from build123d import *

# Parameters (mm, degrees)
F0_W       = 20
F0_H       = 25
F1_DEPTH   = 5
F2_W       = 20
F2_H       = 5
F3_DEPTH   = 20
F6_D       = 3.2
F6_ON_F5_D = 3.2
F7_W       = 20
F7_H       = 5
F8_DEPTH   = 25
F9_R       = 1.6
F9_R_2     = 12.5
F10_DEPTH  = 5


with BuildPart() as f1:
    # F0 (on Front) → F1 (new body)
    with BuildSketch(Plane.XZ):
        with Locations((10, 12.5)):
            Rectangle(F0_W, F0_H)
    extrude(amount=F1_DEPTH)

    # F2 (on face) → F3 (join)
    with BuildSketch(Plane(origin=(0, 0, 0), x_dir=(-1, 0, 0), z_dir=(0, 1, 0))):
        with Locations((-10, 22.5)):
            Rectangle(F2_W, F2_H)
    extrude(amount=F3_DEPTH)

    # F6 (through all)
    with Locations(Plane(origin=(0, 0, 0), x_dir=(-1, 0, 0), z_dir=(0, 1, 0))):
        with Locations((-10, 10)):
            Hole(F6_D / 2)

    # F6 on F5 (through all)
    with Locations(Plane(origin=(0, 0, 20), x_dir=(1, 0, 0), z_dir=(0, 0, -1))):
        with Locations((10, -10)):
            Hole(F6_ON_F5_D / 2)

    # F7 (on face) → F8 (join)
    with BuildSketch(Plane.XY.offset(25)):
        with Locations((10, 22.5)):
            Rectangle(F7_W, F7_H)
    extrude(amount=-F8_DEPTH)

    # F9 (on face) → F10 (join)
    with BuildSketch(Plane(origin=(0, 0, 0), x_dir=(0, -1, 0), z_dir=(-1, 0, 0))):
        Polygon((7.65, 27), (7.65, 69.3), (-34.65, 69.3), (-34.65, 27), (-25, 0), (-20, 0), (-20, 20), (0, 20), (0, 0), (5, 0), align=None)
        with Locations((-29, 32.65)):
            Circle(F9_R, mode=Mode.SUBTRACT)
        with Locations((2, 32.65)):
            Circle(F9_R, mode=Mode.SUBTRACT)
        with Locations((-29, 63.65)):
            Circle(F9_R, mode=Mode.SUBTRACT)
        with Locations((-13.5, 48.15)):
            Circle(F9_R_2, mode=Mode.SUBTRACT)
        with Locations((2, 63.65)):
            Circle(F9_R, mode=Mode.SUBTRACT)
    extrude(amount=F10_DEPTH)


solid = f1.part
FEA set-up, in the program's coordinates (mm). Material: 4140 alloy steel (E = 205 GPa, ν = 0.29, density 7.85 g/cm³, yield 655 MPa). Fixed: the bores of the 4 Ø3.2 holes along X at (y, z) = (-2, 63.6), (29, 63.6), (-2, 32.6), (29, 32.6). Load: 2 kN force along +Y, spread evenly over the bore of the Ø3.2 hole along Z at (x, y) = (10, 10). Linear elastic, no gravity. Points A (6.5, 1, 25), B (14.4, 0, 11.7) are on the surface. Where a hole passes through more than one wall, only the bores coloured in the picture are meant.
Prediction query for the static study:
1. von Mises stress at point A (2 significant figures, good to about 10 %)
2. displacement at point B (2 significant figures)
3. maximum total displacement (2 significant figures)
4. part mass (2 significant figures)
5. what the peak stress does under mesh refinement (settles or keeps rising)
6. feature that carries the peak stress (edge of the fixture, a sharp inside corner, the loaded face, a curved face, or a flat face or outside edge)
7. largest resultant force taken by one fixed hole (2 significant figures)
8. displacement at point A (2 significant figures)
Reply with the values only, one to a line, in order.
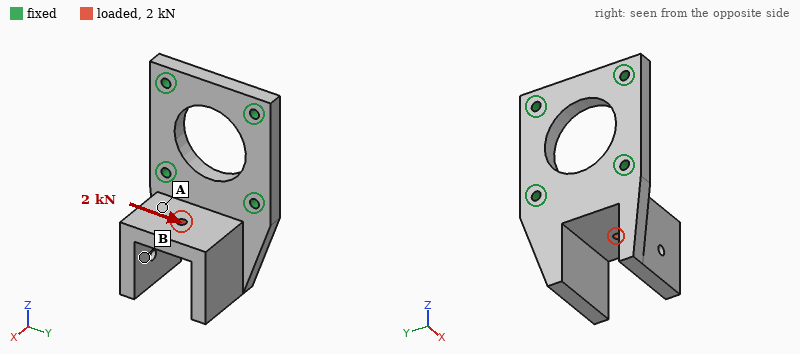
35 MPa
14 µm
19 µm
130 g
keeps rising
edge of the fixture
1.4 kN
8.6 µm
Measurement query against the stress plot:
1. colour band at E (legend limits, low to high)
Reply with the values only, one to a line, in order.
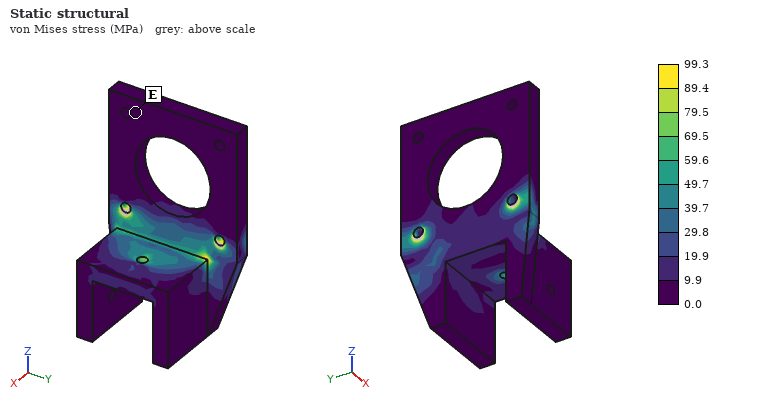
0.0 to 9.9 MPa
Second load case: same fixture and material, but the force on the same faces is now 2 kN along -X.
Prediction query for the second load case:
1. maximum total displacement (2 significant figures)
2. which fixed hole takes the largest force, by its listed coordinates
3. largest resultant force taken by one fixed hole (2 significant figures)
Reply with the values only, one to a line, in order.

65 µm
(-2, 32.6)
1.3 kN
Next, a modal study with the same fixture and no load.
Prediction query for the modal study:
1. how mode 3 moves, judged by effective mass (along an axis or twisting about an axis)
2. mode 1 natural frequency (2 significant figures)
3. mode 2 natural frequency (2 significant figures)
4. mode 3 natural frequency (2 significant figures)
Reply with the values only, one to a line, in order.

along Y
2500 Hz
4900 Hz
6500 Hz
